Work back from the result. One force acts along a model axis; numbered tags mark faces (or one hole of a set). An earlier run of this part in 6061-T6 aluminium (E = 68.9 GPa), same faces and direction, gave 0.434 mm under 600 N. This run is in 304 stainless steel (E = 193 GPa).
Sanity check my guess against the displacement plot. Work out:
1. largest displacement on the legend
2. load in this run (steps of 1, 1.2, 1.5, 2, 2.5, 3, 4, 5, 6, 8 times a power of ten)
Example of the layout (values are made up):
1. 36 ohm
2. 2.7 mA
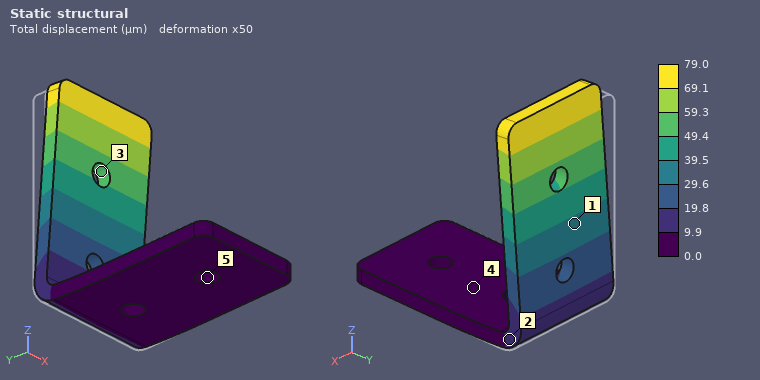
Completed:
1. 79.0 µm
2. 300 N
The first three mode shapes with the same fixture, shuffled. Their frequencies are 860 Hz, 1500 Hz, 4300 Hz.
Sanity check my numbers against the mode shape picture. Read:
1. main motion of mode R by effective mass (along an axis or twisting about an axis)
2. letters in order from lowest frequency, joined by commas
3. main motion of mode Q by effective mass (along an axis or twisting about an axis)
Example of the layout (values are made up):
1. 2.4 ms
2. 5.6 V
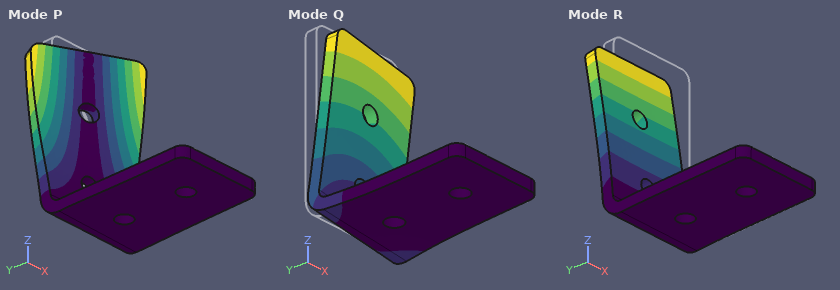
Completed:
1. along Y
2. R, Q, P
3. along X
